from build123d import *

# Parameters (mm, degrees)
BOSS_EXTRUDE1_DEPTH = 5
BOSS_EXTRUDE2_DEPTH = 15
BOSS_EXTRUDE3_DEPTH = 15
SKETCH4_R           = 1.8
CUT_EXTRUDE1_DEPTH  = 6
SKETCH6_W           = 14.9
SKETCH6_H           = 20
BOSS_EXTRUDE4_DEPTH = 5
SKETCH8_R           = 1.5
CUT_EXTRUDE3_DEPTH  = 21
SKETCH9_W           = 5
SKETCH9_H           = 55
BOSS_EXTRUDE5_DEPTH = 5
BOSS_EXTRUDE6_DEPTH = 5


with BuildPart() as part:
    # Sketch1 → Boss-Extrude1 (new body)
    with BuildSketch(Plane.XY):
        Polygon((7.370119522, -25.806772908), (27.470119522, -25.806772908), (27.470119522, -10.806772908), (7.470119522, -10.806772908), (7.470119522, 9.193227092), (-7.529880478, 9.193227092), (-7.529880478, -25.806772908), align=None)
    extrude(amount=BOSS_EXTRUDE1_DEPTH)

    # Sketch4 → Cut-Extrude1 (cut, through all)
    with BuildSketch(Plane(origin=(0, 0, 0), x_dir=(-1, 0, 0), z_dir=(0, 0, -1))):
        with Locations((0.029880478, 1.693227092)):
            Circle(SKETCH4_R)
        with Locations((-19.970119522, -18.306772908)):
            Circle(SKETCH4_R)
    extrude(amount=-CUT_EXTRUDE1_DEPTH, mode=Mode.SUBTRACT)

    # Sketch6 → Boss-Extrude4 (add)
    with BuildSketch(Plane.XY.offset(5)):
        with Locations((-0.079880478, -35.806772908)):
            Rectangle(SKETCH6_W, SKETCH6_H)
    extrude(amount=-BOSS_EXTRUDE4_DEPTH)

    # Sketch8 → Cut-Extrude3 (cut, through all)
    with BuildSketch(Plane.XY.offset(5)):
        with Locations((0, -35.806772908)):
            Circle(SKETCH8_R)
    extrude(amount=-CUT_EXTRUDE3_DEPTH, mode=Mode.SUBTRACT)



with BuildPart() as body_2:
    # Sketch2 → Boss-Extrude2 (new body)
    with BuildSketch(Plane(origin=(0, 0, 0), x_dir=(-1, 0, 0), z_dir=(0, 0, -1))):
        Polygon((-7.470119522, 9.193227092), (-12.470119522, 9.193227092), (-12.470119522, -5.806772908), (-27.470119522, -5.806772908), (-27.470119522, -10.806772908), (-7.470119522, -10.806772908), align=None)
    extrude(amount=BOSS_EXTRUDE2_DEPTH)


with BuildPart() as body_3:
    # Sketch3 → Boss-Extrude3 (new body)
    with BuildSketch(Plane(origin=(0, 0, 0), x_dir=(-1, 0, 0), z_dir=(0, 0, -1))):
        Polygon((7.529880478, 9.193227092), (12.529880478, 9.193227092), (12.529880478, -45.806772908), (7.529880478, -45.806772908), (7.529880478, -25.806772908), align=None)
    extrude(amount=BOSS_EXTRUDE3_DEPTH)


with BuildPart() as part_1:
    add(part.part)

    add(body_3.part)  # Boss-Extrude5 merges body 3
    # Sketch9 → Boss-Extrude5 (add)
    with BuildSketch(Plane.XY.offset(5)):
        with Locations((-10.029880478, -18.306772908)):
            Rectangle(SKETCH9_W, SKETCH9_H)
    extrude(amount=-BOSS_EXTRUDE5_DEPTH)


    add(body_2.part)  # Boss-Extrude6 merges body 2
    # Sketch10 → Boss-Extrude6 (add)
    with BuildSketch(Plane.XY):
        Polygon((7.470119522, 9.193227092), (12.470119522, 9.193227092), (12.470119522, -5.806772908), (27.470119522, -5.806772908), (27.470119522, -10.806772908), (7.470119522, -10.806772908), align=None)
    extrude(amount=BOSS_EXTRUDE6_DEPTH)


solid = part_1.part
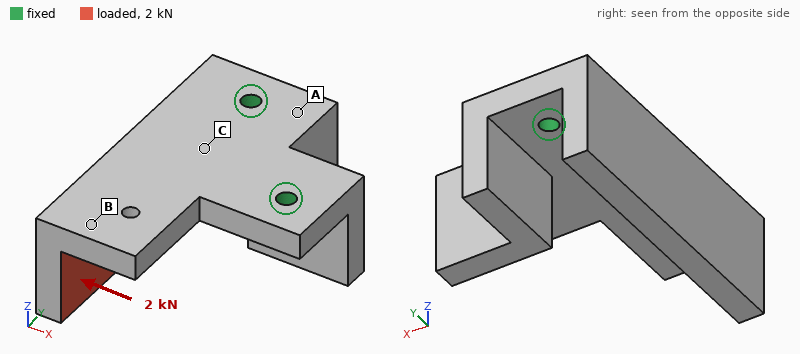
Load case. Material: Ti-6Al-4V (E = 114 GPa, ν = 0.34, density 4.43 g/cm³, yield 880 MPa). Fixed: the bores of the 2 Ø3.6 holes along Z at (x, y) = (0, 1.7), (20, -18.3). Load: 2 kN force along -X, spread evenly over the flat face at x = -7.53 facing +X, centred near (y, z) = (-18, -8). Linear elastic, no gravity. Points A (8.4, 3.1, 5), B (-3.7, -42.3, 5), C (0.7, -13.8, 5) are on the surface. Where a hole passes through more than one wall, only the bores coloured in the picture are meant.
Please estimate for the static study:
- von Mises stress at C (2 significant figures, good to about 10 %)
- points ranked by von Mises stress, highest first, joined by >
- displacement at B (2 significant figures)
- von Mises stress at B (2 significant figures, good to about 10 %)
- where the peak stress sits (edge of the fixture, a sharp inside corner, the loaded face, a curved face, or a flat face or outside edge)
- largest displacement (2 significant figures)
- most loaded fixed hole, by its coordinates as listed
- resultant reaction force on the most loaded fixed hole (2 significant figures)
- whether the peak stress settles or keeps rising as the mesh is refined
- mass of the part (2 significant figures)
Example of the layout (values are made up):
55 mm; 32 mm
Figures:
74 MPa; C > B > A; 0.073 mm; 39 MPa; edge of the fixture; 0.21 mm; (20, -18.3); 1.7 kN; keeps rising; 64 g
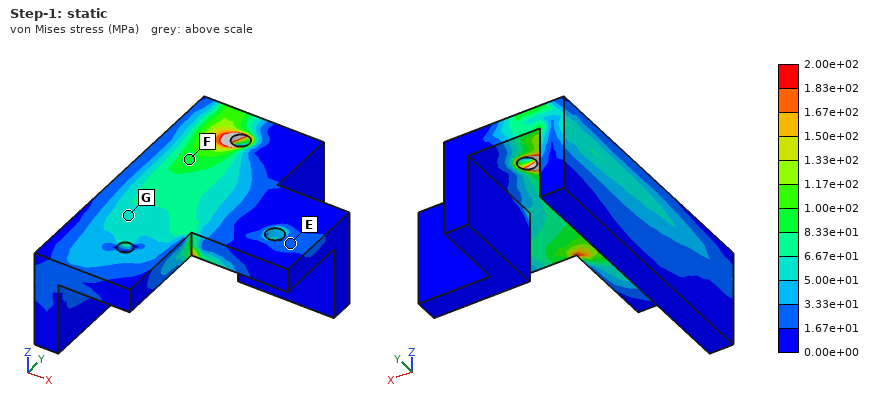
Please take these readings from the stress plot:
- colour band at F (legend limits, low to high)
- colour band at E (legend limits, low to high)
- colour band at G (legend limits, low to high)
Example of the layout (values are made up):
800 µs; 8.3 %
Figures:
8.33e+01 to 1.00e+02 MPa; 1.67e+01 to 3.33e+01 MPa; 5.00e+01 to 6.67e+01 MPa
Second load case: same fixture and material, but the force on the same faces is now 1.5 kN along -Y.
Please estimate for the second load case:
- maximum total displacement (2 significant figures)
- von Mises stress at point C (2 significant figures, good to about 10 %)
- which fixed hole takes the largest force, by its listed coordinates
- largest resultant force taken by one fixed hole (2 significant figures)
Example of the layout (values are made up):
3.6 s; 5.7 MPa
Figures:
0.14 mm; 30 MPa; (0, 1.7); 1.6 kN
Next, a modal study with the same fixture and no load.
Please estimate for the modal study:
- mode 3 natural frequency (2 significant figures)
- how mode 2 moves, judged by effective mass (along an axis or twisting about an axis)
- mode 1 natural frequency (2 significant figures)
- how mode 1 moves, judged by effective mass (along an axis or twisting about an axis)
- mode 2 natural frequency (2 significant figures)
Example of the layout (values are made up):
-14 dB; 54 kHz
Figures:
8800 Hz; along X; 2400 Hz; along Z; 5900 Hz
